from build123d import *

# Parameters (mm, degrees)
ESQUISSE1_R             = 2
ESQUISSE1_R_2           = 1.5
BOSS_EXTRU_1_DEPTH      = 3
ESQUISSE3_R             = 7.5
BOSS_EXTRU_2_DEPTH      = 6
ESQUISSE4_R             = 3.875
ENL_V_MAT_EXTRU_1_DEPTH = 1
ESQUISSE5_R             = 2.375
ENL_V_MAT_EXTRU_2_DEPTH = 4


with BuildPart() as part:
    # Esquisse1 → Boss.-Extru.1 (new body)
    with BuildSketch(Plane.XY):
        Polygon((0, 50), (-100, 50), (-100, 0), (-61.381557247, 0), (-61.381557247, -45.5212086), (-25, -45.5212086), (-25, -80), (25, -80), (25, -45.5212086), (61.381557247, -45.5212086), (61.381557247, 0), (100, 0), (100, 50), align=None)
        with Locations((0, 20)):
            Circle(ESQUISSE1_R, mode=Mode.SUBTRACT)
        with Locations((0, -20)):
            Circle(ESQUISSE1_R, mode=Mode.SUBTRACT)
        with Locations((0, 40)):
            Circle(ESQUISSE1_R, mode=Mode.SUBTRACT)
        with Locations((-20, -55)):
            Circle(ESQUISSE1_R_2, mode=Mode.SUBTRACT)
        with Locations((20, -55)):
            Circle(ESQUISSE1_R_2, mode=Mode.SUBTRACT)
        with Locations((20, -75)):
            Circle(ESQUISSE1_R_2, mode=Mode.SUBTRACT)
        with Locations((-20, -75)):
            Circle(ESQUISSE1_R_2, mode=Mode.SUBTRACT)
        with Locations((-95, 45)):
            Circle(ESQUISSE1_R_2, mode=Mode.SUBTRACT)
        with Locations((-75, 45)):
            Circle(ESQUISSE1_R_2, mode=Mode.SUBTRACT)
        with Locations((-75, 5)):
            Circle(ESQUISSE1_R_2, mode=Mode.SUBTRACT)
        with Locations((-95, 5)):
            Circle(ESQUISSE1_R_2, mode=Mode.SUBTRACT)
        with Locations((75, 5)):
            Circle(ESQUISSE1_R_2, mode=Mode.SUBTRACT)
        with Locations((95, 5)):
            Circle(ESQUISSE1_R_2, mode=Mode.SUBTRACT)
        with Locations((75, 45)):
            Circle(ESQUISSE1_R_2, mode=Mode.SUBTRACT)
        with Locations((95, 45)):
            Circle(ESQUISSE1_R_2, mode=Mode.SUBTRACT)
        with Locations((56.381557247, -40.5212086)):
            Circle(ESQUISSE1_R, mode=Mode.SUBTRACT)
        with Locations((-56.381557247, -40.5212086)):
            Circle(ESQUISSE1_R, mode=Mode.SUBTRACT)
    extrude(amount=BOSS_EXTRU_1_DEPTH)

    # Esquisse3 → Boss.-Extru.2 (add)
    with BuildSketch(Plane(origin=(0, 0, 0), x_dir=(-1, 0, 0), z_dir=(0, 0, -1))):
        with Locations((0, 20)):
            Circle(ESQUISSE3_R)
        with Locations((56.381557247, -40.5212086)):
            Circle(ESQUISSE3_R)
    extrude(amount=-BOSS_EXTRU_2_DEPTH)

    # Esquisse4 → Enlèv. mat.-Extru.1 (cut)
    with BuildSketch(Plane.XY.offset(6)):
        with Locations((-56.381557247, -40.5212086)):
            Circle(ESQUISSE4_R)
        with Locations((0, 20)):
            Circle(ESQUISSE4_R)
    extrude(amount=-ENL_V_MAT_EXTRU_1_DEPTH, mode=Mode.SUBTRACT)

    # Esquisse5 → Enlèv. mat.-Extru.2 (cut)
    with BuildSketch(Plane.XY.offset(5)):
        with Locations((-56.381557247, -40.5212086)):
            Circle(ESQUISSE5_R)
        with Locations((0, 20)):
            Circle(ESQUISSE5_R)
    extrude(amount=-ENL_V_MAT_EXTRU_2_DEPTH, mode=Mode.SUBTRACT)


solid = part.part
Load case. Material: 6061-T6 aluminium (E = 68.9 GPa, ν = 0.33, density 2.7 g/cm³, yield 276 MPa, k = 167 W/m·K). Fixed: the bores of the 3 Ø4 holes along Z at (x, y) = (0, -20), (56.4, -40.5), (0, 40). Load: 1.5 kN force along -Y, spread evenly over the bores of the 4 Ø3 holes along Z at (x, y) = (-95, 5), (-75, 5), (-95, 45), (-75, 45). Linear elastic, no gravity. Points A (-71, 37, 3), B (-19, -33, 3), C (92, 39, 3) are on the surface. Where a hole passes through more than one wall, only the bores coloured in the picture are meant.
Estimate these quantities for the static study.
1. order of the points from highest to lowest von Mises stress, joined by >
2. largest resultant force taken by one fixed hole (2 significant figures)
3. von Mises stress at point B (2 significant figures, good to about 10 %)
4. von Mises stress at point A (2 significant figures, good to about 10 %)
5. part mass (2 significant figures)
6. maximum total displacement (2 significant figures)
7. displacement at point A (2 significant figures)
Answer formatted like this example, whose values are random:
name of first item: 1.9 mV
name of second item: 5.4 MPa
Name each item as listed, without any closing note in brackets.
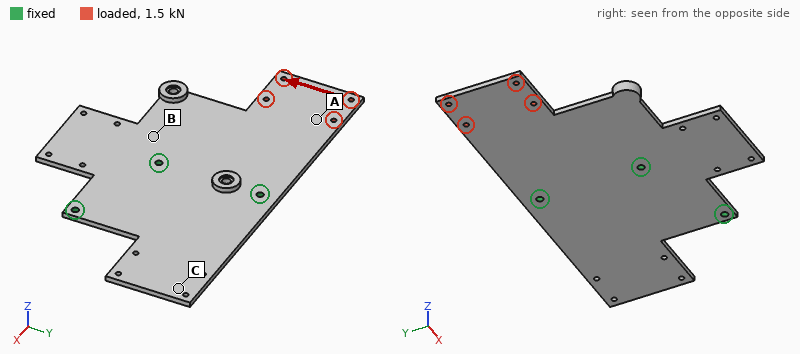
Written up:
order of the points from highest to lowest von Mises stress, joined by >: A > B > C
largest resultant force taken by one fixed hole: 1.9 kN
von Mises stress at point B: 9.8 MPa
von Mises stress at point A: 19 MPa
part mass: 140 g
maximum total displacement: 97 µm
displacement at point A: 57 µm
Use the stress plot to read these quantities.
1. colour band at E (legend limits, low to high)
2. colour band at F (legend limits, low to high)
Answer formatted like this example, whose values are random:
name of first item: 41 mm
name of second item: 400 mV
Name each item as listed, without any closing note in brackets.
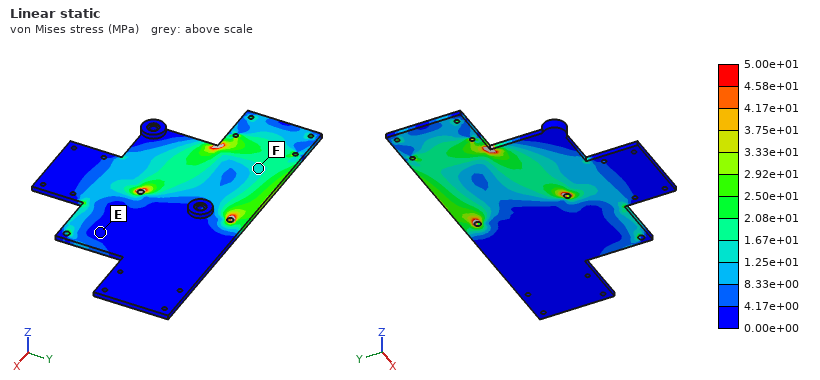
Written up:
colour band at E: 0.00e+00 to 4.17e+00 MPa
colour band at F: 1.25e+01 to 1.67e+01 MPa
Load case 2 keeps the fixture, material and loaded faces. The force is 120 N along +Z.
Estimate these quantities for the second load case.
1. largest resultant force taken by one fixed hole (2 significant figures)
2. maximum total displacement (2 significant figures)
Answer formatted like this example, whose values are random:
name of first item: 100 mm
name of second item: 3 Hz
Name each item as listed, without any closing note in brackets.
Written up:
largest resultant force taken by one fixed hole: 96 N
maximum total displacement: 2.8 mm
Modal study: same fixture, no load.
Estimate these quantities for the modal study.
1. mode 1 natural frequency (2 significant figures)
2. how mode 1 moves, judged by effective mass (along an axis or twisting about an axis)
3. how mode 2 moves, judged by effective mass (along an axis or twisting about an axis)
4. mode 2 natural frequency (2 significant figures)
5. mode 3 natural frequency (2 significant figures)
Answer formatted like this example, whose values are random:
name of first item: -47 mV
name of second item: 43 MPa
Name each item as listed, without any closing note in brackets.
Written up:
mode 1 natural frequency: 290 Hz
how mode 1 moves, judged by effective mass: along Z
how mode 2 moves, judged by effective mass: along Z
mode 2 natural frequency: 380 Hz
mode 3 natural frequency: 720 Hz
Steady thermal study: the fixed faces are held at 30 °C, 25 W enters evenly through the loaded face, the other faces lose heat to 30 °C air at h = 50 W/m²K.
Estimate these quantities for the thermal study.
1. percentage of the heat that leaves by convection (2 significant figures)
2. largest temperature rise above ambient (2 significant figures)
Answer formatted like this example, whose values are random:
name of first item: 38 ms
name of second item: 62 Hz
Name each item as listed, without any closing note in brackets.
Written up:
percentage of the heat that leaves by convection: 61 %
largest temperature rise above ambient: 49 K
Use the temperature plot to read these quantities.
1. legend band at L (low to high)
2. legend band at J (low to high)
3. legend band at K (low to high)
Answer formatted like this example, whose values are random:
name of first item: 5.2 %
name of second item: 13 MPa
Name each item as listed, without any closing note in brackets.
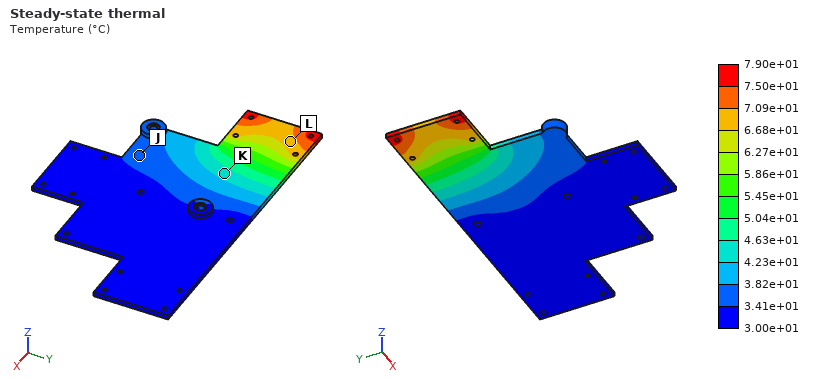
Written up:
legend band at L: 6.68e+01 to 7.09e+01 °C
legend band at J: 3.41e+01 to 3.82e+01 °C
legend band at K: 4.23e+01 to 4.63e+01 °C
